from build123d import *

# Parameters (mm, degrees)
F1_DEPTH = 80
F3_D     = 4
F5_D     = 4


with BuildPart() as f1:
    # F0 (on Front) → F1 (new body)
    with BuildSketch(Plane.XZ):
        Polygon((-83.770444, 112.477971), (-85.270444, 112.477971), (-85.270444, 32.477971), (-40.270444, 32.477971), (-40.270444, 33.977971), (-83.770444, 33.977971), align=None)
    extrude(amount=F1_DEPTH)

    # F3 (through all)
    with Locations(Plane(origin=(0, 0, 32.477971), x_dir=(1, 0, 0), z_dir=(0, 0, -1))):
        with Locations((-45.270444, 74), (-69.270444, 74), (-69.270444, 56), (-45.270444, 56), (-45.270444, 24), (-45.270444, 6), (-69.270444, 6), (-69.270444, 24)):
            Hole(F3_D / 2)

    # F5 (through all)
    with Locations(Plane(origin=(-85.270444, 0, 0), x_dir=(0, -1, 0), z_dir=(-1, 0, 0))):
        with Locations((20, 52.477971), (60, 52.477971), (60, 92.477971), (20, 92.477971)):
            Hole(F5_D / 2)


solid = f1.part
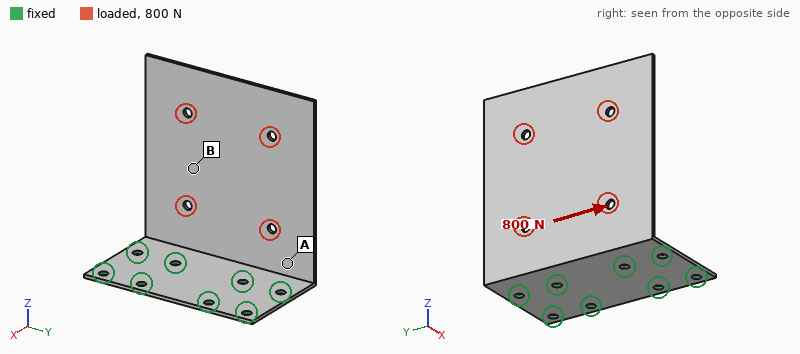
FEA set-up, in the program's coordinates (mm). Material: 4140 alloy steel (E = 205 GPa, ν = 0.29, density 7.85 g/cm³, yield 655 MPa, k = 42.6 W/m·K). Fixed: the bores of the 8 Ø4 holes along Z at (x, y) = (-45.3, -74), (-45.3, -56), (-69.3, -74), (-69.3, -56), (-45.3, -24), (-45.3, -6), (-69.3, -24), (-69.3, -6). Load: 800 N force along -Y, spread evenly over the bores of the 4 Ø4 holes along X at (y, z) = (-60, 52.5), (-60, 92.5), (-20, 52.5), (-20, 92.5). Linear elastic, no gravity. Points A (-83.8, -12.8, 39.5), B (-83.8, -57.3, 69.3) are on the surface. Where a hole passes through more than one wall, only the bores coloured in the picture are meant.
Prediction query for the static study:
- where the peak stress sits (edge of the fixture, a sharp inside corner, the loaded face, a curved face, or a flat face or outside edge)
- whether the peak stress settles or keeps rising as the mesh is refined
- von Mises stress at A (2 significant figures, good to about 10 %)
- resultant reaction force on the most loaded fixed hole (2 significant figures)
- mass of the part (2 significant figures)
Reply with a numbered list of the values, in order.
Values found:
1. edge of the fixture
2. keeps rising
3. 140 MPa
4. 440 N
5. 110 g
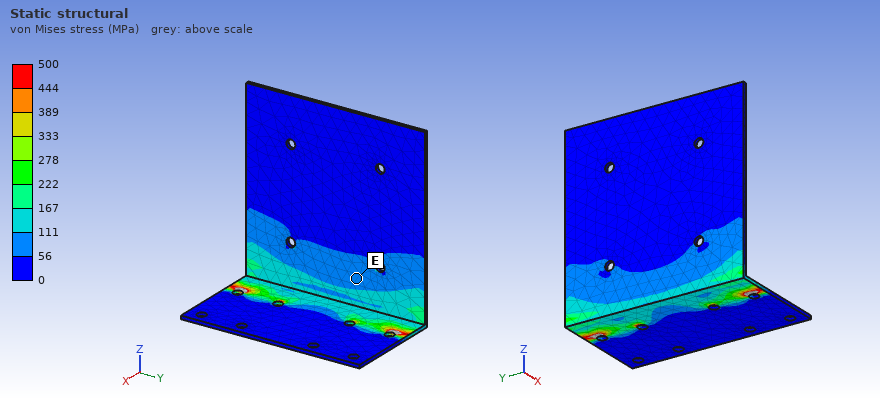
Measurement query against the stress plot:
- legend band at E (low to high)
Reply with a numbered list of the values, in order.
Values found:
1. 56 to 111 MPa
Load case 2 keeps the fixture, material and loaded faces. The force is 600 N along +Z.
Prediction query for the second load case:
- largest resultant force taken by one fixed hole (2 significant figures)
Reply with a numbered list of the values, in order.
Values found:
1. 190 N
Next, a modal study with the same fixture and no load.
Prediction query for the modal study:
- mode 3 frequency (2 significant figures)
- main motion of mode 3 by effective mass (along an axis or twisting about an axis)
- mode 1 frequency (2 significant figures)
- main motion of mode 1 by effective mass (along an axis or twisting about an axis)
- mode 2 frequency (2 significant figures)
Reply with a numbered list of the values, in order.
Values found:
1. 810 Hz
2. along Y
3. 150 Hz
4. along X
5. 430 Hz
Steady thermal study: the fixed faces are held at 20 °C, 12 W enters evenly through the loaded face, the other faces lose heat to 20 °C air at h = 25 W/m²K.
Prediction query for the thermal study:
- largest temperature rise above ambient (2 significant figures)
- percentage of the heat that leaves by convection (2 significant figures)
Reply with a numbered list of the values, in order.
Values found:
1. 44 K
2. 74 %
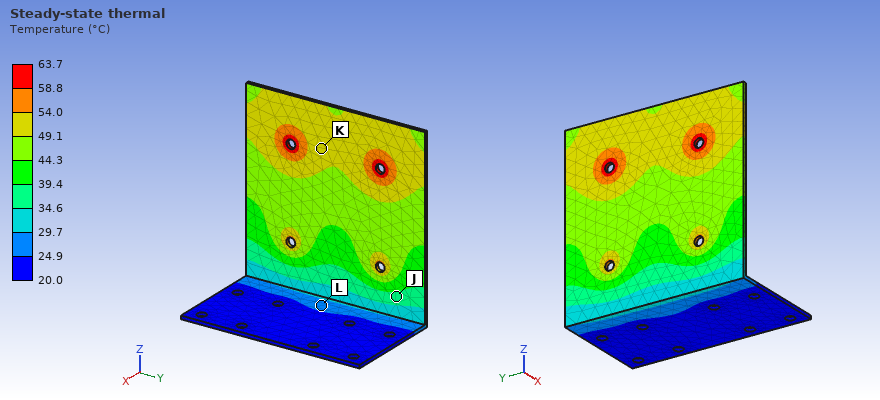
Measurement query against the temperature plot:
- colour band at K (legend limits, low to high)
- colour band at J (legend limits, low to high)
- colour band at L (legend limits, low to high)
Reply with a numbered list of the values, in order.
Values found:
1. 49.1 to 54.0 °C
2. 34.6 to 39.4 °C
3. 24.9 to 29.7 °C
